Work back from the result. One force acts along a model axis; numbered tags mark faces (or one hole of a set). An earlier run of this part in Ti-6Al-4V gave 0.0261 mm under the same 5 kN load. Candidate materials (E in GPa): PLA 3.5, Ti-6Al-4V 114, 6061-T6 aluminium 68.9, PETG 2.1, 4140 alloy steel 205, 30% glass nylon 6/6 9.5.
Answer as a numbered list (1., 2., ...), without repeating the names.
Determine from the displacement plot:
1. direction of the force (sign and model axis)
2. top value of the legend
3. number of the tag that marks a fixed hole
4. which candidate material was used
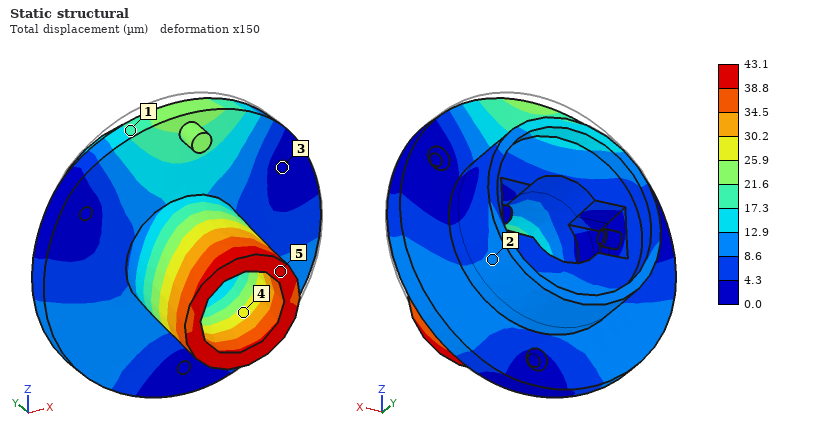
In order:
1. -Z
2. 43.1 µm
3. 3
4. 6061-T6 aluminium
